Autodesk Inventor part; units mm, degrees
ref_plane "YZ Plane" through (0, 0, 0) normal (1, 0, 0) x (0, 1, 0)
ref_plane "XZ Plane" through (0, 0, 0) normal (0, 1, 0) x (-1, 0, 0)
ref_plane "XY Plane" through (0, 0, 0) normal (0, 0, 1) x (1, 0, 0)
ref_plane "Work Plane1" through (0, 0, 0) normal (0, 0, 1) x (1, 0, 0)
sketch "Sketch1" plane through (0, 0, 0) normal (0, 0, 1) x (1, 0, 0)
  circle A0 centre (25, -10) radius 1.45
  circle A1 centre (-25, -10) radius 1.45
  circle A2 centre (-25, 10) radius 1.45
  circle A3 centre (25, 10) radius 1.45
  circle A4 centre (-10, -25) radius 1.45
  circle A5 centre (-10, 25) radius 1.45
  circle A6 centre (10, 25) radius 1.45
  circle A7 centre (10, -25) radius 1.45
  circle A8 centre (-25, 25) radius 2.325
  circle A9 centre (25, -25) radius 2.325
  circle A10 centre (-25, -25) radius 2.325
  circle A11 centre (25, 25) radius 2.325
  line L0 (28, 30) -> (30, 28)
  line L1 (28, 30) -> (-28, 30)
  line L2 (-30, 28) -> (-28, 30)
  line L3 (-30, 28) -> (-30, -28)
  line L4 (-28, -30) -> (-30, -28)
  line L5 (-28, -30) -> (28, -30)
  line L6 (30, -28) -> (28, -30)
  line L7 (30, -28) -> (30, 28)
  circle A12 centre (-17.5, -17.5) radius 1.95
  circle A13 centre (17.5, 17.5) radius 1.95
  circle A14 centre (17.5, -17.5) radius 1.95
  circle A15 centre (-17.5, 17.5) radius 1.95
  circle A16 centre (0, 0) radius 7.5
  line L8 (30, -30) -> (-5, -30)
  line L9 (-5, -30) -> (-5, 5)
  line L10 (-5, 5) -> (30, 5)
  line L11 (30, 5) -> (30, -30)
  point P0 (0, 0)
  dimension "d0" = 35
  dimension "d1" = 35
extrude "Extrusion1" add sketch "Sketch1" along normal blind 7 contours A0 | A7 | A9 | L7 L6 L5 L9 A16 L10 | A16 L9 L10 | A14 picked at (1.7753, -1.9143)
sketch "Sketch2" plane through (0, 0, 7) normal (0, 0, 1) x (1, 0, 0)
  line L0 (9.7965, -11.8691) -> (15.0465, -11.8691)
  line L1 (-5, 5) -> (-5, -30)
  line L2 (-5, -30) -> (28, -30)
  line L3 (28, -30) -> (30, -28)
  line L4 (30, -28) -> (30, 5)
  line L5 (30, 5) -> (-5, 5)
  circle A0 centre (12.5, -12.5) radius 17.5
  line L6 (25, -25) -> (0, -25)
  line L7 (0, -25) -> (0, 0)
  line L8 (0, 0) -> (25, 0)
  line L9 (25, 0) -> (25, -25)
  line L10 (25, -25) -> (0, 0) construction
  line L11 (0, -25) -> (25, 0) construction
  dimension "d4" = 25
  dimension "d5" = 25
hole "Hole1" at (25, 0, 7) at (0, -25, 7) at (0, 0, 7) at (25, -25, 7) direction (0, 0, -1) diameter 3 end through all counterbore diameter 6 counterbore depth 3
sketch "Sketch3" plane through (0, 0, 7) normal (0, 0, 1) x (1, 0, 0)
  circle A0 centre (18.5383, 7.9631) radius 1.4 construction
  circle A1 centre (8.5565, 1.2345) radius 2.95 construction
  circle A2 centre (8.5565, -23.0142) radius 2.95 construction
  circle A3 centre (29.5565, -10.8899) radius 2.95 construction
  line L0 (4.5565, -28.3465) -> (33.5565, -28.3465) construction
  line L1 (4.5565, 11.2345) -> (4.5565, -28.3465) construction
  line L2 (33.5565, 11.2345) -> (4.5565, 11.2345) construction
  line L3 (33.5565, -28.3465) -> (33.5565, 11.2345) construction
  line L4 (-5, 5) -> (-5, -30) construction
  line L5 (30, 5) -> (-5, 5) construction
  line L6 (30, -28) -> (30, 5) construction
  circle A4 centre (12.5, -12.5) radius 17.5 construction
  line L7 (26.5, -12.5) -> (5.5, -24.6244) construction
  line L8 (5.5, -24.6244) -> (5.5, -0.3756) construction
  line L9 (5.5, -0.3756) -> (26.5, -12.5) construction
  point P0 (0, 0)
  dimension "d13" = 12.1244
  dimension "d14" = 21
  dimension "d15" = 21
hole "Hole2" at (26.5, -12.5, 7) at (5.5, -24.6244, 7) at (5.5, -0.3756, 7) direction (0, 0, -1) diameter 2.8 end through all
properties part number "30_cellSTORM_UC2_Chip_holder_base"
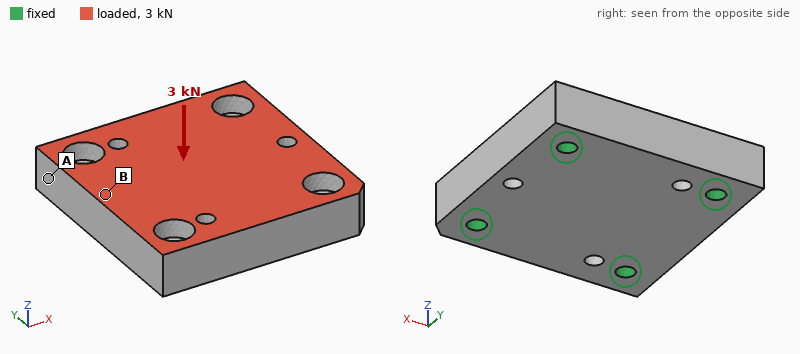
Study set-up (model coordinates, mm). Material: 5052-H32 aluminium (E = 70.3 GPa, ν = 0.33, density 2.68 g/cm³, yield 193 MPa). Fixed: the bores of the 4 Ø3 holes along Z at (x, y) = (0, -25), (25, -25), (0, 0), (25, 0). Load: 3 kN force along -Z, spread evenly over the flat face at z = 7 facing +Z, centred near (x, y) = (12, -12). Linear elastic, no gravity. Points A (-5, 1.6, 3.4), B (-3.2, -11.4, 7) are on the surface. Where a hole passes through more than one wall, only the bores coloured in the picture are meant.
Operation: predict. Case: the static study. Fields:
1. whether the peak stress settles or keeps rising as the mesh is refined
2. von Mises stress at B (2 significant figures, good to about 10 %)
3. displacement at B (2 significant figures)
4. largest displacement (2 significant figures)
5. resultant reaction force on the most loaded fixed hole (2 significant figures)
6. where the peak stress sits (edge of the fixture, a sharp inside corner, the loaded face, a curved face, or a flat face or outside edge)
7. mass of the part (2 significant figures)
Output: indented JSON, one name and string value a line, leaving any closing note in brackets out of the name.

{
  "whether the peak stress settles or keeps rising as the mesh is refined": "keeps rising",
  "von Mises stress at B": "15 MPa",
  "displacement at B": "4.5 µm",
  "largest displacement": "7.3 µm",
  "resultant reaction force on the most loaded fixed hole": "810 N",
  "where the peak stress sits": "edge of the fixture",
  "mass of the part": "21 g"
}
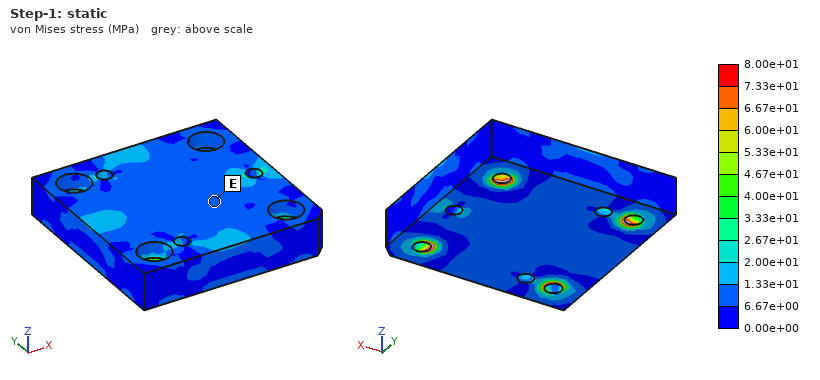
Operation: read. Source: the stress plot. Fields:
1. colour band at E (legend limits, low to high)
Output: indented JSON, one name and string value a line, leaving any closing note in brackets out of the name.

{
  "colour band at E": "6.67e+00 to 1.33e+01 MPa"
}
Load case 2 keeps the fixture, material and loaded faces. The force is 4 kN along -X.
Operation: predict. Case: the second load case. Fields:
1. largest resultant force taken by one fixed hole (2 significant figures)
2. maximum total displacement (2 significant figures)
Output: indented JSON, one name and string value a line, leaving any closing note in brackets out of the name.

{
  "largest resultant force taken by one fixed hole": "1.1 kN",
  "maximum total displacement": "7.1 µm"
}
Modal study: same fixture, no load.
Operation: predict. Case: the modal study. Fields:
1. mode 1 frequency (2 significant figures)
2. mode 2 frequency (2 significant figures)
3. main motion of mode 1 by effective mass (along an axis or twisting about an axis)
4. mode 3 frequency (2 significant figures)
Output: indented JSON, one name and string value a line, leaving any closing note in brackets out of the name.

{
  "mode 1 frequency": "26 kHz",
  "mode 2 frequency": "36 kHz",
  "main motion of mode 1 by effective mass": "along Z",
  "mode 3 frequency": "36 kHz"
}
